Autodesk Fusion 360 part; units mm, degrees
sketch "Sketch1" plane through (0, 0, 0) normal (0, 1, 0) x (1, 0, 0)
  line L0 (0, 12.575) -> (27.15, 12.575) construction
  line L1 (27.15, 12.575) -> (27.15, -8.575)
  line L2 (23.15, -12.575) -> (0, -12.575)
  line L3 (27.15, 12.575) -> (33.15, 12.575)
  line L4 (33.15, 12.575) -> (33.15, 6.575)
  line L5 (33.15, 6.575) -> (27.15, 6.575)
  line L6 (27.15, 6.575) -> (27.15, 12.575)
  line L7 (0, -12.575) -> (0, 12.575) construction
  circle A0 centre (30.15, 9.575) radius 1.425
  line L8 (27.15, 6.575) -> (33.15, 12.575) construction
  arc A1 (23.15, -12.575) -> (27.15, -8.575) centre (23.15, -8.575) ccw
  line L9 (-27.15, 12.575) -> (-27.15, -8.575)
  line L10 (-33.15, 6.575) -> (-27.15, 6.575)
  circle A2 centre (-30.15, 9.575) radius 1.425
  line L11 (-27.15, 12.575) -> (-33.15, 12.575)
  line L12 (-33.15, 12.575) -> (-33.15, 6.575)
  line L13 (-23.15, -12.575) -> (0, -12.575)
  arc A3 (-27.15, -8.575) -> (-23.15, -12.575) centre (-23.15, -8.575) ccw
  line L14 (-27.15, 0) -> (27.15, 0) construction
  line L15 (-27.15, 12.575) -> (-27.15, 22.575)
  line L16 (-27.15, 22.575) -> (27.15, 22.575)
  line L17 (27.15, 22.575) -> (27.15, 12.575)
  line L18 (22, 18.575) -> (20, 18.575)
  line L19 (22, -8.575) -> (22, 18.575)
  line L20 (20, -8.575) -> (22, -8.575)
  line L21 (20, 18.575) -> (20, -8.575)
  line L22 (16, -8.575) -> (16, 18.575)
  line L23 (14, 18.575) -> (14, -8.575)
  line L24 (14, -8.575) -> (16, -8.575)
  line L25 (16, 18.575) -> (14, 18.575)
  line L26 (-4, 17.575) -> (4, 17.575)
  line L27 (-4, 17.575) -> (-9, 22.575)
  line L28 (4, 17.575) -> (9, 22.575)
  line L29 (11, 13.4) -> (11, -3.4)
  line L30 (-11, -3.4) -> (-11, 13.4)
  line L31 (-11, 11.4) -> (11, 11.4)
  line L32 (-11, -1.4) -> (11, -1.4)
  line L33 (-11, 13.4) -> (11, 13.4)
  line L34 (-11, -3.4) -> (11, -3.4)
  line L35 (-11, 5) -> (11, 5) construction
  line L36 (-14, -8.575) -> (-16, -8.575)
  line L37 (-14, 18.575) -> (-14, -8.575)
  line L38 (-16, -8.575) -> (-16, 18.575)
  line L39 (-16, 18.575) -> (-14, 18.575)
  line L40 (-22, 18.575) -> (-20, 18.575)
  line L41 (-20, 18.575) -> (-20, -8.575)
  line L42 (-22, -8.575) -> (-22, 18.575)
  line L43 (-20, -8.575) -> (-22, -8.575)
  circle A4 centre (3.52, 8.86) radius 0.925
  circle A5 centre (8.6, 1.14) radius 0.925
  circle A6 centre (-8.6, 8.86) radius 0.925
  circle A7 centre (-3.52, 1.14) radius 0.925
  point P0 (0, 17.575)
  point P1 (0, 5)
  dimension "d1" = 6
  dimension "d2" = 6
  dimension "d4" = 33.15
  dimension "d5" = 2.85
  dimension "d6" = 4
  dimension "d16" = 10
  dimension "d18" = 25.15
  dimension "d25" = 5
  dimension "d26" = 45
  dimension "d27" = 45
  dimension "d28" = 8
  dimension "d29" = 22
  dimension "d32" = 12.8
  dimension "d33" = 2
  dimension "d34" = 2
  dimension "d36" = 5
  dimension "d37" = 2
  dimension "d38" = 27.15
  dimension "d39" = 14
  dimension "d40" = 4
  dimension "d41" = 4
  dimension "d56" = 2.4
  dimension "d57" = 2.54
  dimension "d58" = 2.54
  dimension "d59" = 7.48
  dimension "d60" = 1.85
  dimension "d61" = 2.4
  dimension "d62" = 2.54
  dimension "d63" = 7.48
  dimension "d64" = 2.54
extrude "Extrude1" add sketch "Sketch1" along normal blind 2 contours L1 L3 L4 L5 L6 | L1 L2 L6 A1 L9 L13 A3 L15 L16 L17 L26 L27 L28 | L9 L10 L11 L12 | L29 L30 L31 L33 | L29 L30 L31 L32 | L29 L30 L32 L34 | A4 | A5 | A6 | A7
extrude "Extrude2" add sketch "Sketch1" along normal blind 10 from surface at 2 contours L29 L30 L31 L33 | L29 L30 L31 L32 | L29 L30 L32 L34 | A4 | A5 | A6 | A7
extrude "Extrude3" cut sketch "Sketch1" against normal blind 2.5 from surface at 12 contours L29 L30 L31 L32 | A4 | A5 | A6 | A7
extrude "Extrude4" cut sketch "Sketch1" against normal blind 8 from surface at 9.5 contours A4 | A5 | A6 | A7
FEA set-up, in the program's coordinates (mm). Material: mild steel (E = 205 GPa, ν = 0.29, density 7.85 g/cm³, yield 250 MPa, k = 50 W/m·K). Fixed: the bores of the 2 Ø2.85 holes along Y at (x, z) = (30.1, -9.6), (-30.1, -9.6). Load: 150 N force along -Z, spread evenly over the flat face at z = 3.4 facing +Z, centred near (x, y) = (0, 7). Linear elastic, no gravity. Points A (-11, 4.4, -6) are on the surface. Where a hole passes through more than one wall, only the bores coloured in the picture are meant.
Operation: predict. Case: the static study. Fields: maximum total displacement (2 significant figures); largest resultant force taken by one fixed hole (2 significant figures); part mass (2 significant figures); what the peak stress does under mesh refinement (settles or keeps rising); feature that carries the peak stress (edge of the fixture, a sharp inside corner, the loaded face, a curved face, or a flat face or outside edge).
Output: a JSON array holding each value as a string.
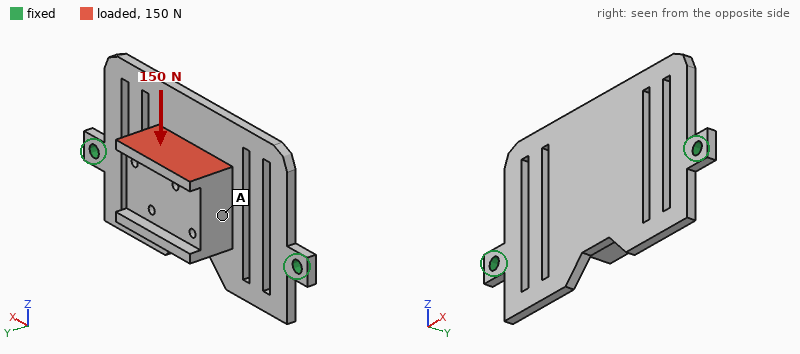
["85 µm", "75 N", "49 g", "keeps rising", "edge of the fixture"]
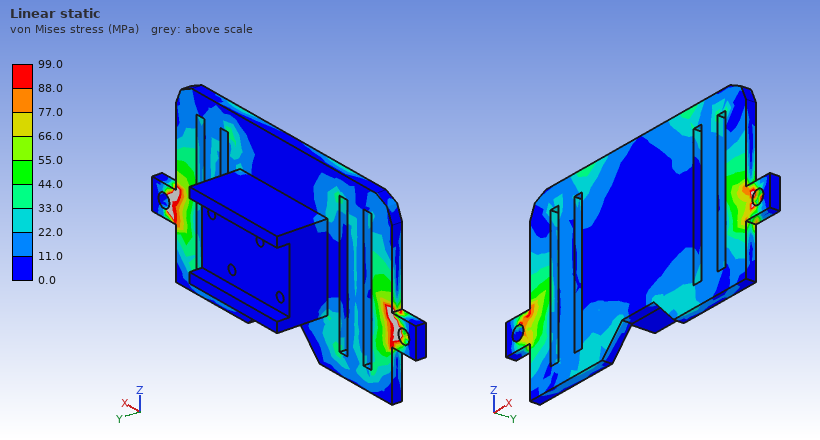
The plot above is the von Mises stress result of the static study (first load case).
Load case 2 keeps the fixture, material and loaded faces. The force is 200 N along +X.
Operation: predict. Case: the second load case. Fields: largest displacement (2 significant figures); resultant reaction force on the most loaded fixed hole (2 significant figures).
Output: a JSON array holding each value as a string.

["26 µm", "110 N"]
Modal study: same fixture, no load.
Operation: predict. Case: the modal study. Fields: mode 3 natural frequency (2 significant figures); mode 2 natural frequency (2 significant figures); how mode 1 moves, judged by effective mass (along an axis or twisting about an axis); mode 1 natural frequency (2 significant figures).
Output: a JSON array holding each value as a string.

["2500 Hz", "1600 Hz", "along Y", "900 Hz"]
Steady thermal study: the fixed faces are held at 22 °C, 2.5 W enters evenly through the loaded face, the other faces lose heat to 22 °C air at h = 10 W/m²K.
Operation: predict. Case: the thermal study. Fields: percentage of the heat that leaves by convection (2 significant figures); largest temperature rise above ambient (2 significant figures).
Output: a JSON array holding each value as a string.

["41 %", "31 K"]
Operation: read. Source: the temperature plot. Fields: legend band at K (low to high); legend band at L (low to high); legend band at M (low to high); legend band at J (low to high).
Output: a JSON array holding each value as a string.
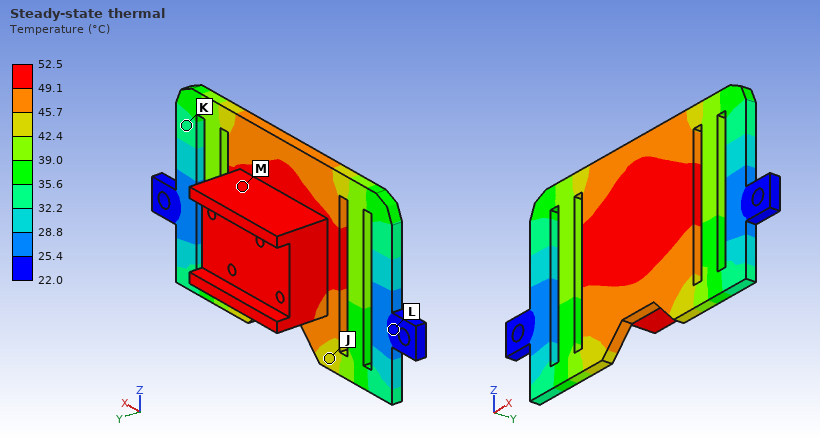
["32.2 to 35.6 °C", "22.0 to 25.4 °C", "49.1 to 52.5 °C", "42.4 to 45.7 °C"]
